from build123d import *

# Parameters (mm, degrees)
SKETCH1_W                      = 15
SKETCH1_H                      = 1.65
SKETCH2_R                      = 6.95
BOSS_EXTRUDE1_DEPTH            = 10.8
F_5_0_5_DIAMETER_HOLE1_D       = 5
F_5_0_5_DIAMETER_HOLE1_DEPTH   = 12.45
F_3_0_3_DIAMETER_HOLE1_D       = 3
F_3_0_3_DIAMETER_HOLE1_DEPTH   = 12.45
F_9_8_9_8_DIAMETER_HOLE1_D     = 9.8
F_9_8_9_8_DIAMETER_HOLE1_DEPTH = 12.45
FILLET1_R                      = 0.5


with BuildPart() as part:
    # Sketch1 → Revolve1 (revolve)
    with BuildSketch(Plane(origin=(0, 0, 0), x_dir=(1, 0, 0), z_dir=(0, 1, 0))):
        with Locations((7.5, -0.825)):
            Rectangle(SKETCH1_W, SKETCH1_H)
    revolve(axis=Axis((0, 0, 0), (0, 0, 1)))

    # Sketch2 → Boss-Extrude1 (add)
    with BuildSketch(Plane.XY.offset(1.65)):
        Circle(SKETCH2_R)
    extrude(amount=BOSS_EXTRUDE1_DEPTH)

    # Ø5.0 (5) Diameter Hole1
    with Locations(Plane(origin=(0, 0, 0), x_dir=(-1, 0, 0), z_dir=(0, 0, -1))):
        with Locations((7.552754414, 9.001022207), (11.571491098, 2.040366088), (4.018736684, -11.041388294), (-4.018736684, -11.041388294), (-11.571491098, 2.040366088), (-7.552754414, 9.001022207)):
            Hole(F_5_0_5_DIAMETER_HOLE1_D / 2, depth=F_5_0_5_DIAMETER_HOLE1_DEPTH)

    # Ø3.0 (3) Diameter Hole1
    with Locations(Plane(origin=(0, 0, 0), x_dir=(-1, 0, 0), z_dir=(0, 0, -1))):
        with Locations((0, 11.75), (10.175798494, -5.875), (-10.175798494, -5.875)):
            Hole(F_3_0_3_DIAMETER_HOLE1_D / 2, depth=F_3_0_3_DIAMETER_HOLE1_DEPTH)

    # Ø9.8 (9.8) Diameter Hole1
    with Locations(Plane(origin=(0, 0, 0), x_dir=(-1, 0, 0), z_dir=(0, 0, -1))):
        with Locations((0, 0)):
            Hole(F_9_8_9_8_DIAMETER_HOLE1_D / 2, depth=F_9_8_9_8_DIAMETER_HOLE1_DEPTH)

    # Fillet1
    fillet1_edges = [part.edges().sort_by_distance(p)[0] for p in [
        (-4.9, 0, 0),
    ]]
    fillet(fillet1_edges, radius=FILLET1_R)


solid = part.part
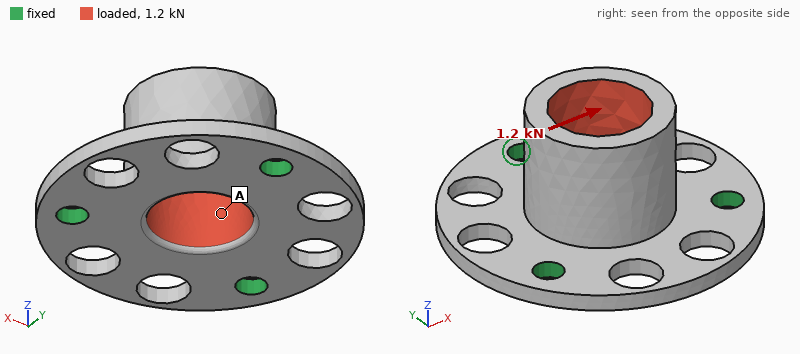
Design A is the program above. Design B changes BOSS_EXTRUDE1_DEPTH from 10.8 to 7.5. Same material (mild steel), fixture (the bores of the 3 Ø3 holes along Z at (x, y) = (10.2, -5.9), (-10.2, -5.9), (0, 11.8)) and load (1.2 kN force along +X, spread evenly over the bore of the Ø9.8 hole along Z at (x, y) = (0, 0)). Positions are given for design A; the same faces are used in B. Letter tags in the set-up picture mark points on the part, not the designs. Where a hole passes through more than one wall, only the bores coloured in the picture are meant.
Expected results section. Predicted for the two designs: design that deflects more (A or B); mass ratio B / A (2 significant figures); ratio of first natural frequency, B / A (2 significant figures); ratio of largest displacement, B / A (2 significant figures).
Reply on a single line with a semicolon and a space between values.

A; 0.85; 1.2; 0.61
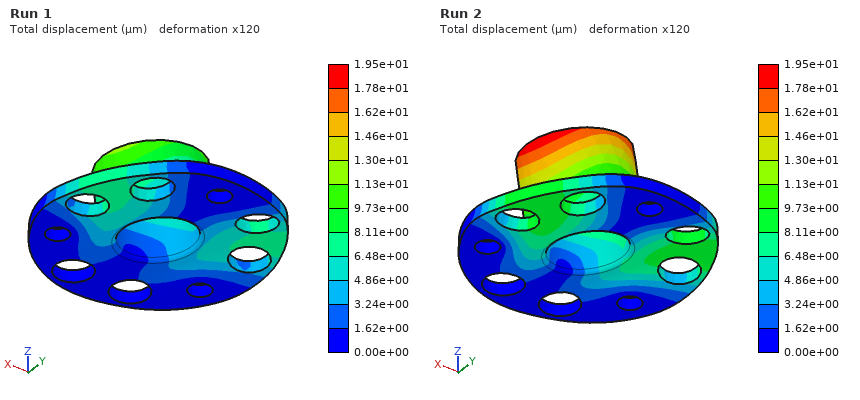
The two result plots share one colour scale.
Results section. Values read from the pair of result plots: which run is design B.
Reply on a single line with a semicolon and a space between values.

Run 1
